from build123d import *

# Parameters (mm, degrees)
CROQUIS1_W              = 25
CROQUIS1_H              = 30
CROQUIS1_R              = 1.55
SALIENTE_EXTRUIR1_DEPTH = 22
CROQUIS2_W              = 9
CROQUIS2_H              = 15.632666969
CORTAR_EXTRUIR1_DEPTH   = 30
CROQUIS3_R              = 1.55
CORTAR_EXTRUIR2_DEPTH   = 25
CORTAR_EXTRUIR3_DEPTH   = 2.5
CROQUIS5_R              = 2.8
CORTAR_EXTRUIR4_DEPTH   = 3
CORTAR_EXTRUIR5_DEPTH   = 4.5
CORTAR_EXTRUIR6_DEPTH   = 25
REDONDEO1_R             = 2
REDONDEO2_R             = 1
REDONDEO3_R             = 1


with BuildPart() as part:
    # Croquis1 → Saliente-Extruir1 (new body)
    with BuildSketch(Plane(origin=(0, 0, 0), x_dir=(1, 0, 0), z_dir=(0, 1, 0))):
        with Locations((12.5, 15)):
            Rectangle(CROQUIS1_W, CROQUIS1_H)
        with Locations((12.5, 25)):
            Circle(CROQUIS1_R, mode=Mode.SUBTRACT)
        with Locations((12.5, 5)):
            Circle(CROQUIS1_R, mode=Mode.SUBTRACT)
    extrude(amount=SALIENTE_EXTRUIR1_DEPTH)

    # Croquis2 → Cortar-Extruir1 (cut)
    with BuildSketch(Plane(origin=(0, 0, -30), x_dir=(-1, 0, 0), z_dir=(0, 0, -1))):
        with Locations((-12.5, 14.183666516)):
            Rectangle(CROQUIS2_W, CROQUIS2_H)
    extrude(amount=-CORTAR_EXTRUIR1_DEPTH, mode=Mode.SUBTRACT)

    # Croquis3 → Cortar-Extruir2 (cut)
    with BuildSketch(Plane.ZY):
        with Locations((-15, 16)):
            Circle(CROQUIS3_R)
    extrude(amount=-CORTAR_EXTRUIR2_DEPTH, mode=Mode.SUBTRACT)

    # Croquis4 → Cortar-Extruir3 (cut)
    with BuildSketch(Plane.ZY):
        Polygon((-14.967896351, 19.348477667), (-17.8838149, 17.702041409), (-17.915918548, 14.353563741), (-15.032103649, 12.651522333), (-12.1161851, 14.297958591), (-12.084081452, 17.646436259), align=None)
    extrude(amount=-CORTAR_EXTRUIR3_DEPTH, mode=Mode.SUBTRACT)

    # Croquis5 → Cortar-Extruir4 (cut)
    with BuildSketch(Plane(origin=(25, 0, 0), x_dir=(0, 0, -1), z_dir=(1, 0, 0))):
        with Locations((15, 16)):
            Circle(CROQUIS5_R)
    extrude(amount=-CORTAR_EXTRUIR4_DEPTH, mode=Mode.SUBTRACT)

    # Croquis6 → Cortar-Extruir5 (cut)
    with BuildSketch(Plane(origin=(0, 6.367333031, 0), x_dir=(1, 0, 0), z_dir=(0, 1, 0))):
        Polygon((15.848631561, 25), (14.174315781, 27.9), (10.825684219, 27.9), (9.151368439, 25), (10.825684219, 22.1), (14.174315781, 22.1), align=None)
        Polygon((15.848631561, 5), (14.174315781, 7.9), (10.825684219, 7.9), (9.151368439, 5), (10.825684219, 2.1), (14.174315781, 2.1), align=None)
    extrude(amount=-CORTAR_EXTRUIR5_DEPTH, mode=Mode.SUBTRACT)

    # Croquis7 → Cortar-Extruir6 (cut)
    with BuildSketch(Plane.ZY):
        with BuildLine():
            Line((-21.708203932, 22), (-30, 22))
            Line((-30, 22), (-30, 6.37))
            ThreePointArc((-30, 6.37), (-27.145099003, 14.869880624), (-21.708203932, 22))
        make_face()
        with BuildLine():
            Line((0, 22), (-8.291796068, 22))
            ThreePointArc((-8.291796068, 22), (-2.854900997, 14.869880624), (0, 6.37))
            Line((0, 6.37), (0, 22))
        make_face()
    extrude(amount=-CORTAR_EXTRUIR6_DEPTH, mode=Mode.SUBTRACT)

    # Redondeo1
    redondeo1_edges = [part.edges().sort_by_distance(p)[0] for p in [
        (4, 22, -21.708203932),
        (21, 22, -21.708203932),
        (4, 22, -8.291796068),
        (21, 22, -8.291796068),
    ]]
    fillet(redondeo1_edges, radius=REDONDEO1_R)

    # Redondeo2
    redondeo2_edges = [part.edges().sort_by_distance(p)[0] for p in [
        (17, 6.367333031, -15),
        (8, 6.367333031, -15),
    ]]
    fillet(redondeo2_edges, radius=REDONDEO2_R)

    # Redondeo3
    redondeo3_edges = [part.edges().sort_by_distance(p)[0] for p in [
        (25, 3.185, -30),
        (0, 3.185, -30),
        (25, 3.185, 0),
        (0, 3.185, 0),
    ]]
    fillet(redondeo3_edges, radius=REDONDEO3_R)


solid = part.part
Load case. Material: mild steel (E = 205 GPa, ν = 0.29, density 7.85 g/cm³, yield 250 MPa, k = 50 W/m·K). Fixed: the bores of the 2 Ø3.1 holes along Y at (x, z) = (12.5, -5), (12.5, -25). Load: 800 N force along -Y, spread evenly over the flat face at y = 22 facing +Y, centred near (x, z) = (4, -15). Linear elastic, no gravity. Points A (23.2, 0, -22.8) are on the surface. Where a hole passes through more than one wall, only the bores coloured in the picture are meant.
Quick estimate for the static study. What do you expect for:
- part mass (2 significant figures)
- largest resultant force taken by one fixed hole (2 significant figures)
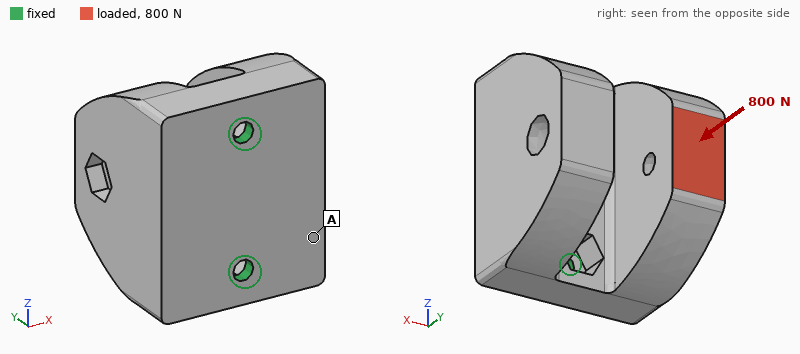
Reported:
80 g
410 N
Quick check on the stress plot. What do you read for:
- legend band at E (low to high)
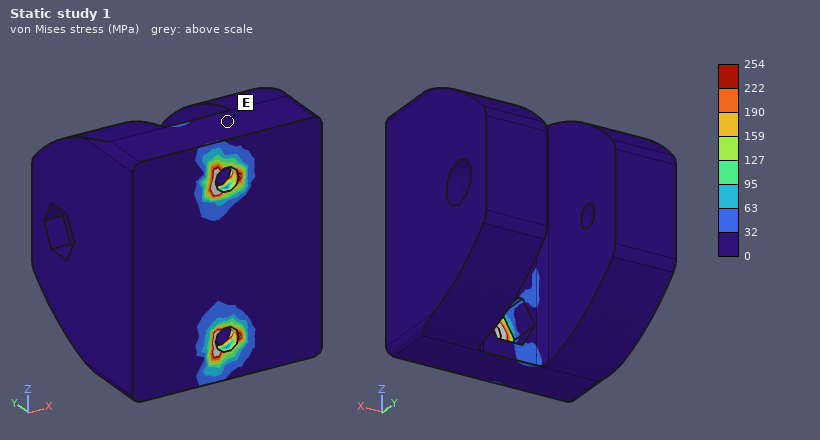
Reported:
0 to 32 MPa
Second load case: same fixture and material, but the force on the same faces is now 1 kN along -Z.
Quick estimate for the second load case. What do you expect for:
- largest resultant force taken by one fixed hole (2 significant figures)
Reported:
1.2 kN
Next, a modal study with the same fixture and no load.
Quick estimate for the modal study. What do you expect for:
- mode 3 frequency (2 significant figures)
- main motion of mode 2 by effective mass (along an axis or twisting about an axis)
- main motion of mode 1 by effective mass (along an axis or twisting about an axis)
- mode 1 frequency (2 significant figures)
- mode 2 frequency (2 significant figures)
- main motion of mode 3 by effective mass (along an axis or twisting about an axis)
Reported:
12 kHz
along Y
along X
2900 Hz
9500 Hz
along Z
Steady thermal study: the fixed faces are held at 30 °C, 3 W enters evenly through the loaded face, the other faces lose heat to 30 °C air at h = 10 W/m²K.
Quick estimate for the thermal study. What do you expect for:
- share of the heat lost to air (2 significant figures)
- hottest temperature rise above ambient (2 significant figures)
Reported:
5.4 %
12 K
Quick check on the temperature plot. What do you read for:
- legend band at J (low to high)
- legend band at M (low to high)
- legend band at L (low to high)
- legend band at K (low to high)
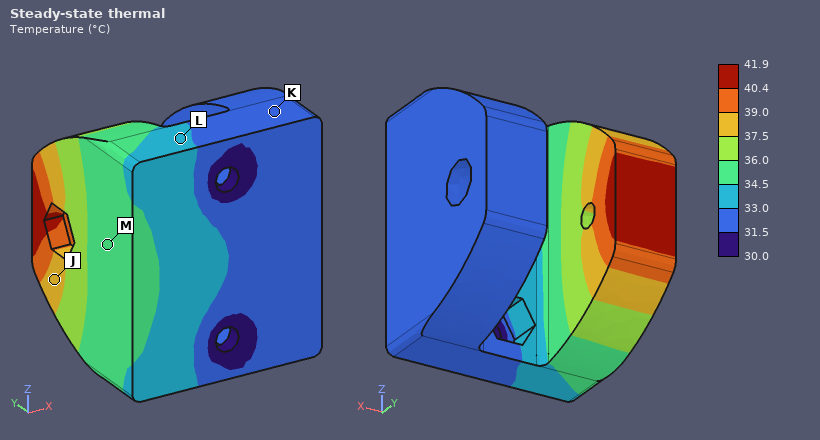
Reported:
37.5 to 39.0 °C
34.5 to 36.0 °C
33.0 to 34.5 °C
31.5 to 33.0 °C
